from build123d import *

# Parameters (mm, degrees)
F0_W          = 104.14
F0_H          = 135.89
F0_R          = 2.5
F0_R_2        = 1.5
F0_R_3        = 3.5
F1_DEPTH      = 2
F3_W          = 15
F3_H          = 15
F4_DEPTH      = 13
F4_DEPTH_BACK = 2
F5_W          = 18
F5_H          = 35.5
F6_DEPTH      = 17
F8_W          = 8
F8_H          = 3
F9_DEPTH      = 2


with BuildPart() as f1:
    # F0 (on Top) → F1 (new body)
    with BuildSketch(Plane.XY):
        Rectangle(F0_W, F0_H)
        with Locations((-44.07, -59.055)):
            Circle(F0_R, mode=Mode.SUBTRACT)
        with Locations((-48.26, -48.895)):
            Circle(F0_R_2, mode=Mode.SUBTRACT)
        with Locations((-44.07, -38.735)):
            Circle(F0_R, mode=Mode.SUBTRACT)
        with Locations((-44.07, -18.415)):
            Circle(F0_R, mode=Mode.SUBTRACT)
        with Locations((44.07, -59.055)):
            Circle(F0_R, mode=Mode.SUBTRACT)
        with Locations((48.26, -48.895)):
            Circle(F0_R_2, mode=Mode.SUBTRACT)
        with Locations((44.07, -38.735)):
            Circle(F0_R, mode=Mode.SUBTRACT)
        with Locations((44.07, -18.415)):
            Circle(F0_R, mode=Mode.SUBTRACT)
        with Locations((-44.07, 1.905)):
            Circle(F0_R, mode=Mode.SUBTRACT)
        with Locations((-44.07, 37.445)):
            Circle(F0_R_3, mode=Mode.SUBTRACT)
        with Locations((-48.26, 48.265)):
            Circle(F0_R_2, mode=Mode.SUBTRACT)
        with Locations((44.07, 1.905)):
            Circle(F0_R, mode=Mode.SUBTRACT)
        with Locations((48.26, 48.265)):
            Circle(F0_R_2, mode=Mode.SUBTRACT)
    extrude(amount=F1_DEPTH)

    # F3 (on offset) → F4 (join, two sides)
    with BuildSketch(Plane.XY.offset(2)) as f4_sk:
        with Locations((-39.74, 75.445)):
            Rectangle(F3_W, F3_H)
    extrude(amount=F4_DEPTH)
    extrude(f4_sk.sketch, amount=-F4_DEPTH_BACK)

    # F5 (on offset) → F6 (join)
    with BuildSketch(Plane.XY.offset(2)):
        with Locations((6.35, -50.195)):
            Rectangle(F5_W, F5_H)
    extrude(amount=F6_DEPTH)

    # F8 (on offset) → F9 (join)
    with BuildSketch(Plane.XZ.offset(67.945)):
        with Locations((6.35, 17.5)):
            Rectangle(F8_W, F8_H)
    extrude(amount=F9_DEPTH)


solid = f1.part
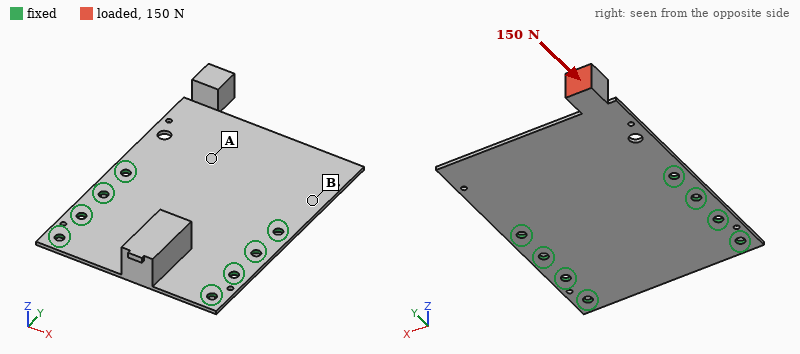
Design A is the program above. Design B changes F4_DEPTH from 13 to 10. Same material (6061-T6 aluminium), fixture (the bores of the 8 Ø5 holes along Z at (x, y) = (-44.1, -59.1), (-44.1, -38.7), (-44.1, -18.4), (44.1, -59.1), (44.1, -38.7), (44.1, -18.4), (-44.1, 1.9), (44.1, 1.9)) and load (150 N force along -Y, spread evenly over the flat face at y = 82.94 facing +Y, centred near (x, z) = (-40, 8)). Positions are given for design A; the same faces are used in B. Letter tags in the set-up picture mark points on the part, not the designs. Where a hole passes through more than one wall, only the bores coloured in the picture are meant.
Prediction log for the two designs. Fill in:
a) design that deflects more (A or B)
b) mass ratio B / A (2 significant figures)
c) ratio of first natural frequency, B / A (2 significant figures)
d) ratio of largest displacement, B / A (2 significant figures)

A
0.98
1.1
0.75
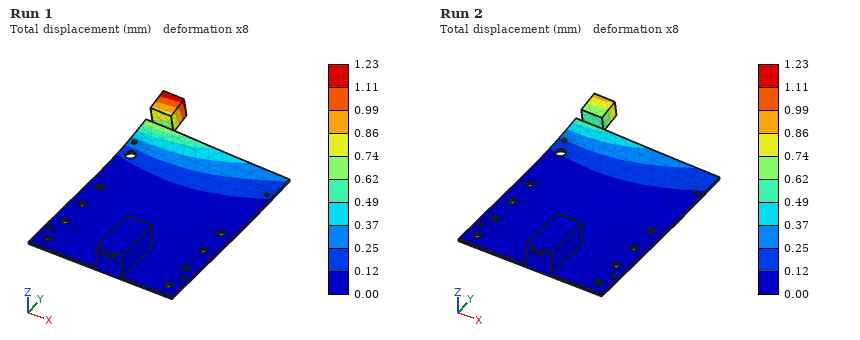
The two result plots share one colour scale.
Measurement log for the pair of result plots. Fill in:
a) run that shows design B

Run 2
